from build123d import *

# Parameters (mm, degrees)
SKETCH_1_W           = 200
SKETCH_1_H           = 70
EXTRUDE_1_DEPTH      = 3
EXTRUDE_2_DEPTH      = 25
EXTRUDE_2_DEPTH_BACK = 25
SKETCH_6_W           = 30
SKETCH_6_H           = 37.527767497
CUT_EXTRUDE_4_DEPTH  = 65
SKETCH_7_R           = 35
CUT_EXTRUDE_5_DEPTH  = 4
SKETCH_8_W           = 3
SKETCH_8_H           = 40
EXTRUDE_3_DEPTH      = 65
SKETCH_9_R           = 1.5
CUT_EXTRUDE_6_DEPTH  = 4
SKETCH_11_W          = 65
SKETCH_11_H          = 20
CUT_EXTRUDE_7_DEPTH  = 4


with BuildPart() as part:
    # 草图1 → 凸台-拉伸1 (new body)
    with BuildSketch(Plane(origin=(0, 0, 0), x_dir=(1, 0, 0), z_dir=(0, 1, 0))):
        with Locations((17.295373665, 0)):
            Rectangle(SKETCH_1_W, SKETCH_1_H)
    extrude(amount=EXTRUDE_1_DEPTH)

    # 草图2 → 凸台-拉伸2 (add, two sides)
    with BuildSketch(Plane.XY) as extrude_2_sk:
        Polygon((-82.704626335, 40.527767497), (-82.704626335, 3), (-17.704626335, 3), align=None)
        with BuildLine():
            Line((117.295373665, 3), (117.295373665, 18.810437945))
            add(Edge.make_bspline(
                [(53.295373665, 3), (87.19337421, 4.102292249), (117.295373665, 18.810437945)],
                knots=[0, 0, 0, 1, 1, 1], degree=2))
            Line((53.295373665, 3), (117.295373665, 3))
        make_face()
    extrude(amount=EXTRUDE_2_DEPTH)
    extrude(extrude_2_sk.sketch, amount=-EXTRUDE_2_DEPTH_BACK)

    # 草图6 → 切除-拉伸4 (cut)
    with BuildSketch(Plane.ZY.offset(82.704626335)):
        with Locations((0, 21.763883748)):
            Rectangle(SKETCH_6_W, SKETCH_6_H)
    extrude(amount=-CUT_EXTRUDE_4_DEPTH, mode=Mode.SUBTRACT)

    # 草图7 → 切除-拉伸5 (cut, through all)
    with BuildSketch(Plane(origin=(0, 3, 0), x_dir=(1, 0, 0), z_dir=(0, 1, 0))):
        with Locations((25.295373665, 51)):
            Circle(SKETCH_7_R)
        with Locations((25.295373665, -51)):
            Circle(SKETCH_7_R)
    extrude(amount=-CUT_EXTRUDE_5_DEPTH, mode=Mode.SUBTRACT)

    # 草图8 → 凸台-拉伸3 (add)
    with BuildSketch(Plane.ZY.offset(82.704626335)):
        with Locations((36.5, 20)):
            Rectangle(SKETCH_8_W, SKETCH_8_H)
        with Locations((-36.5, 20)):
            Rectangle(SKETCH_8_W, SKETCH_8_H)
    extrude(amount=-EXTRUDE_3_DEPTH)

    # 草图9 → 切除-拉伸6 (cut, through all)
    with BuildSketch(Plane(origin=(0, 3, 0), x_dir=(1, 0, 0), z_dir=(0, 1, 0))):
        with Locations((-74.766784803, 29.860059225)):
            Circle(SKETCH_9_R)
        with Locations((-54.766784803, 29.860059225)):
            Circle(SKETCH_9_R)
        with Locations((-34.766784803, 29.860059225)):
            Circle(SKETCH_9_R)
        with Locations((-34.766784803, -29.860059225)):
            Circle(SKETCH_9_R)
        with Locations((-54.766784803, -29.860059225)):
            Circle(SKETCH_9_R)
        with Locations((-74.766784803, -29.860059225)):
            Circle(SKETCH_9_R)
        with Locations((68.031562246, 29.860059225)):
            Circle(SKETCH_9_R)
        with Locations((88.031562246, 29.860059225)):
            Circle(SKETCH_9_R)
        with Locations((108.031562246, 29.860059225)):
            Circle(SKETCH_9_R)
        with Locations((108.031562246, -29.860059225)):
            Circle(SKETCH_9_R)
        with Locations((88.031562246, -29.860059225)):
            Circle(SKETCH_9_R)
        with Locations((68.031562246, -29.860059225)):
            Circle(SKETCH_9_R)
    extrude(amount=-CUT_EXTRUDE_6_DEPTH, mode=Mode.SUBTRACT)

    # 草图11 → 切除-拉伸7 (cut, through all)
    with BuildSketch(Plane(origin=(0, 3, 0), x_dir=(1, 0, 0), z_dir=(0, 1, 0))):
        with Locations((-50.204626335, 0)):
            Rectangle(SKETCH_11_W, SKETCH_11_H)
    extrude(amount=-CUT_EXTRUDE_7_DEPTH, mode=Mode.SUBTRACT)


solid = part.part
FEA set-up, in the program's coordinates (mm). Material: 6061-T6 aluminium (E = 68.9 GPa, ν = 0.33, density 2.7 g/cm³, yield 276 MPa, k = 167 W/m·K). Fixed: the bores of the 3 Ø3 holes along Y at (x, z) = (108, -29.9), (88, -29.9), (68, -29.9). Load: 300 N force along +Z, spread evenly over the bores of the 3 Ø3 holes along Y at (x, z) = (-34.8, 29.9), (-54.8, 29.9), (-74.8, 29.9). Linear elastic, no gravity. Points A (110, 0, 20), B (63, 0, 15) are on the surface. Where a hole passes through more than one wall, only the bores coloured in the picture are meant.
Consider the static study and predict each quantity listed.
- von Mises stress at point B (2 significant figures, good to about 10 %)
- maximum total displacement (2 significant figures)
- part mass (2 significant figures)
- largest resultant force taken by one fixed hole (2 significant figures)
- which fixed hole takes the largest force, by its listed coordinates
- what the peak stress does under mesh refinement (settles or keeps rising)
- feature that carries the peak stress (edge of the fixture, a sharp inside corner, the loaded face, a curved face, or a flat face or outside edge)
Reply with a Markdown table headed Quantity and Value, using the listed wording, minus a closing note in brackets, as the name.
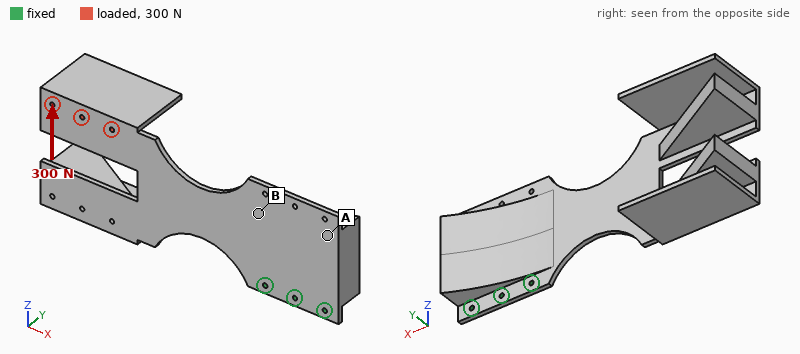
| Quantity | Value |
|---|---|
| von Mises stress at point B | 13 MPa |
| maximum total displacement | 0.42 mm |
| part mass | 240 g |
| largest resultant force taken by one fixed hole | 1.2 kN |
| which fixed hole takes the largest force, by its listed coordinates | (68, -29.9) |
| what the peak stress does under mesh refinement | keeps rising |
| feature that carries the peak stress | edge of the fixture |
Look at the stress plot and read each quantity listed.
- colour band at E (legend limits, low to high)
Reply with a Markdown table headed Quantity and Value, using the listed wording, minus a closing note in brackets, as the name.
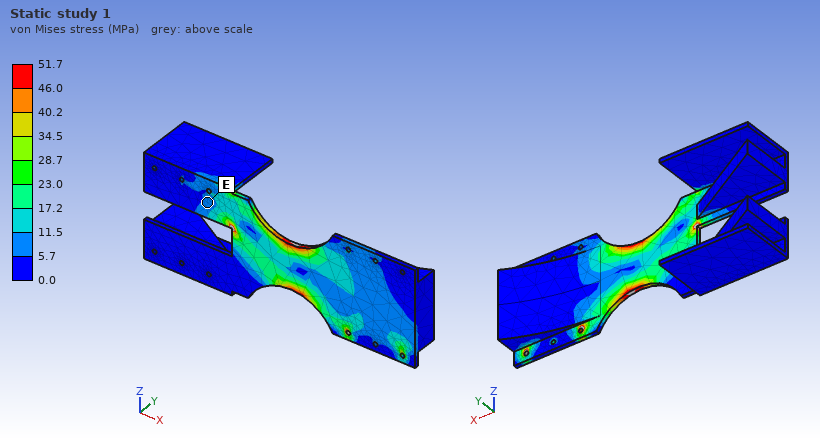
| Quantity | Value |
|---|---|
| colour band at E | 5.7 to 11.5 MPa |
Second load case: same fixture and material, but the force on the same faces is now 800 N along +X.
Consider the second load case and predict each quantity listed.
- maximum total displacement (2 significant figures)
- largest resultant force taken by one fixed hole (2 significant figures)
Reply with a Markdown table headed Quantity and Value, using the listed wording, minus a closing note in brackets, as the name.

| Quantity | Value |
|---|---|
| maximum total displacement | 0.43 mm |
| largest resultant force taken by one fixed hole | 1.2 kN |
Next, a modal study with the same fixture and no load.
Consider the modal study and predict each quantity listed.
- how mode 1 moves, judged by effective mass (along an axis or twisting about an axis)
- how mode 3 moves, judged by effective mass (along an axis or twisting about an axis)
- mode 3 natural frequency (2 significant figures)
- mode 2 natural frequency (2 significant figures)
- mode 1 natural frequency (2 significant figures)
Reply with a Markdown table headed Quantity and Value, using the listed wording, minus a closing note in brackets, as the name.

| Quantity | Value |
|---|---|
| how mode 1 moves, judged by effective mass | along Y |
| how mode 3 moves, judged by effective mass | along Z |
| mode 3 natural frequency | 280 Hz |
| mode 2 natural frequency | 110 Hz |
| mode 1 natural frequency | 44 Hz |
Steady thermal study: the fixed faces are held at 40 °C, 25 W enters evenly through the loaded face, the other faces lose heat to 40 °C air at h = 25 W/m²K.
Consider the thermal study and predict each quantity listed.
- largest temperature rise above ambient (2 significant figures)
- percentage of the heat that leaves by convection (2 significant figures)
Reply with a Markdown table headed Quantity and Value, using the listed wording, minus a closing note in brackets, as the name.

| Quantity | Value |
|---|---|
| largest temperature rise above ambient | 56 K |
| percentage of the heat that leaves by convection | 83 % |
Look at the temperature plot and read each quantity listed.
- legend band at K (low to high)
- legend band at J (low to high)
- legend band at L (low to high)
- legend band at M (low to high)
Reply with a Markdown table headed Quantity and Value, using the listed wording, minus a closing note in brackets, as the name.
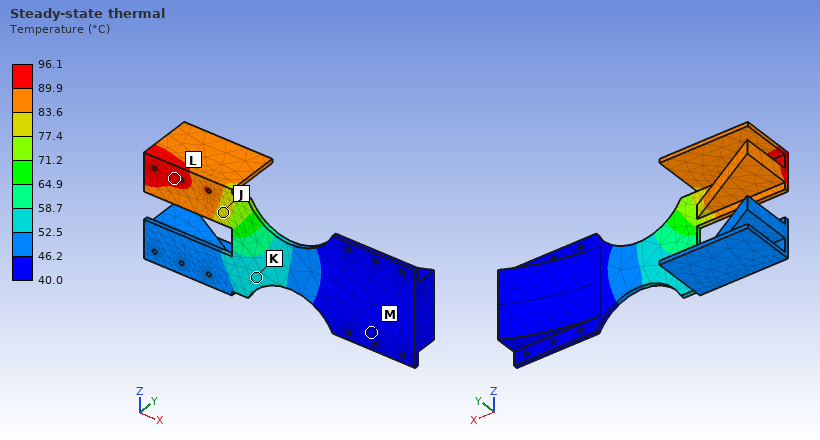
| Quantity | Value |
|---|---|
| legend band at K | 52.5 to 58.7 °C |
| legend band at J | 77.4 to 83.6 °C |
| legend band at L | 89.9 to 96.1 °C |
| legend band at M | 40.0 to 46.2 °C |
